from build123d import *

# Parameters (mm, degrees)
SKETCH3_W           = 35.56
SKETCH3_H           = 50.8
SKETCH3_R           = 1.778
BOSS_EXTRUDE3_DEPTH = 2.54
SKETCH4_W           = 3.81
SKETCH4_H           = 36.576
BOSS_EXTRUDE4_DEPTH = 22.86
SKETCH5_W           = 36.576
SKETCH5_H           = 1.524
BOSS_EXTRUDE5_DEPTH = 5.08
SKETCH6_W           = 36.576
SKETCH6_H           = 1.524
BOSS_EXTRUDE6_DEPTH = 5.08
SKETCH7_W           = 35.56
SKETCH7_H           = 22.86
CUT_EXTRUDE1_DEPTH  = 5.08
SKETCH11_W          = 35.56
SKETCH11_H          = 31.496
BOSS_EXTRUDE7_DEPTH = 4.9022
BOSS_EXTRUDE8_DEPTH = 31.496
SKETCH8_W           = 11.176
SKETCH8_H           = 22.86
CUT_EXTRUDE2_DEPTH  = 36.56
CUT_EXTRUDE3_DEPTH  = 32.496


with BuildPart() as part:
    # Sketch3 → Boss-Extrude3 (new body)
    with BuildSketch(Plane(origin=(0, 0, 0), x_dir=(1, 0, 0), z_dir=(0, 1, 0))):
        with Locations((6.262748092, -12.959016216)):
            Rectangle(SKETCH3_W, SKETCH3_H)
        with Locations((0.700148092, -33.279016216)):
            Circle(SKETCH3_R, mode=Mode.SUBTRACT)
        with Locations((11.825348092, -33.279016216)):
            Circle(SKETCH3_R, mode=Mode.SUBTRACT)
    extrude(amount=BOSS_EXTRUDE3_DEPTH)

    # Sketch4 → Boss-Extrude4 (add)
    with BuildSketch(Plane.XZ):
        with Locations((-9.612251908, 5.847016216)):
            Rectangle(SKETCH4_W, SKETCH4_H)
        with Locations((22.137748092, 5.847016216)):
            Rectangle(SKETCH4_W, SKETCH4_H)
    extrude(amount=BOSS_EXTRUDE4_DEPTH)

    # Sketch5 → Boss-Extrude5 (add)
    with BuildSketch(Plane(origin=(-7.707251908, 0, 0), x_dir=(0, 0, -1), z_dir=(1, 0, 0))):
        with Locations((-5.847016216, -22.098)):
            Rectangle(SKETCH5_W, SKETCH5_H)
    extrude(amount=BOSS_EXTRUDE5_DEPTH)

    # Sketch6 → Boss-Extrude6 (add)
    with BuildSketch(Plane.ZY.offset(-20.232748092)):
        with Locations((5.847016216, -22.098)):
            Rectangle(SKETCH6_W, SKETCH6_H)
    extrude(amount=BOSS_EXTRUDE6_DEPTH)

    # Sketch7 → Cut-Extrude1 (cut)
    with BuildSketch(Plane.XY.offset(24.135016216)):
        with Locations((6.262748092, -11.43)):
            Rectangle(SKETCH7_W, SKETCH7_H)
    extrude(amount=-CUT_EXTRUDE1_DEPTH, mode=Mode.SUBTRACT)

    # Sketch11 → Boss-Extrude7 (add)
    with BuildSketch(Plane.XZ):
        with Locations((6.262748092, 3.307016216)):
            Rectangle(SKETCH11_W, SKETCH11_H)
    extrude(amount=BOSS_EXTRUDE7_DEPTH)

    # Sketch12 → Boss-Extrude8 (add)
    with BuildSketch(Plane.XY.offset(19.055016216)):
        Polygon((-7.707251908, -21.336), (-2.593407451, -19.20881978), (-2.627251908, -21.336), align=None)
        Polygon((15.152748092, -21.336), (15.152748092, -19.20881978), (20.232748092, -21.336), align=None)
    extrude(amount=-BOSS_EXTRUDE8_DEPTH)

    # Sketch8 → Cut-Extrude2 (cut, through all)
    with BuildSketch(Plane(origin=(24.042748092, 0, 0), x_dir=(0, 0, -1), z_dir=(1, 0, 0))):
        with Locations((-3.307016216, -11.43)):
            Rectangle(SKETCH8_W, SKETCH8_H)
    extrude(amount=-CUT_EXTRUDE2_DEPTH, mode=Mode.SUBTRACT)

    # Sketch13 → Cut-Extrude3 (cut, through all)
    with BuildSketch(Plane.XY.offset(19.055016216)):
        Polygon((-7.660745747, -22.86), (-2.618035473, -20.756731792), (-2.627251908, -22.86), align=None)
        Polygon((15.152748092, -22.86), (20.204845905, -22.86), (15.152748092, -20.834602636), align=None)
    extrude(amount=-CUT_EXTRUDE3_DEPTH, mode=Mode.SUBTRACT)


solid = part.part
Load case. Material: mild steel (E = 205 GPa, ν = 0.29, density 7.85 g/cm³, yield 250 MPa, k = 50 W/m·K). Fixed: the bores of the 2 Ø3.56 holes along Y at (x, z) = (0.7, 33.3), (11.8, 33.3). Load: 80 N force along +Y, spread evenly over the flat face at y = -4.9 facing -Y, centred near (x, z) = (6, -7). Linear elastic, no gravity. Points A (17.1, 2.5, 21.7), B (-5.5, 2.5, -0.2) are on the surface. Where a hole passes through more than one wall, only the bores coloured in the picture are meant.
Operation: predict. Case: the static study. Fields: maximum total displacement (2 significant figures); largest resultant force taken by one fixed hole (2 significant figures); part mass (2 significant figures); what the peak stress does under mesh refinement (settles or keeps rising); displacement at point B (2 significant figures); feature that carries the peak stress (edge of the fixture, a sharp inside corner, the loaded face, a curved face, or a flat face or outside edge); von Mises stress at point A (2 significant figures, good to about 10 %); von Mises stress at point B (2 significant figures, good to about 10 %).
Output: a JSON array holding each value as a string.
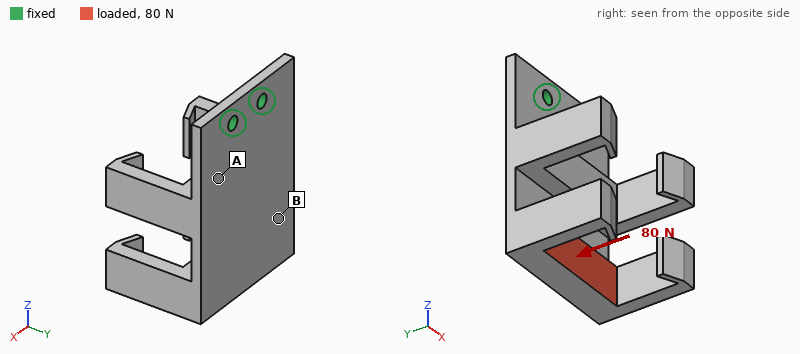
["0.21 mm", "40 N", "88 g", "keeps rising", "0.11 mm", "edge of the fixture", "55 MPa", "14 MPa"]
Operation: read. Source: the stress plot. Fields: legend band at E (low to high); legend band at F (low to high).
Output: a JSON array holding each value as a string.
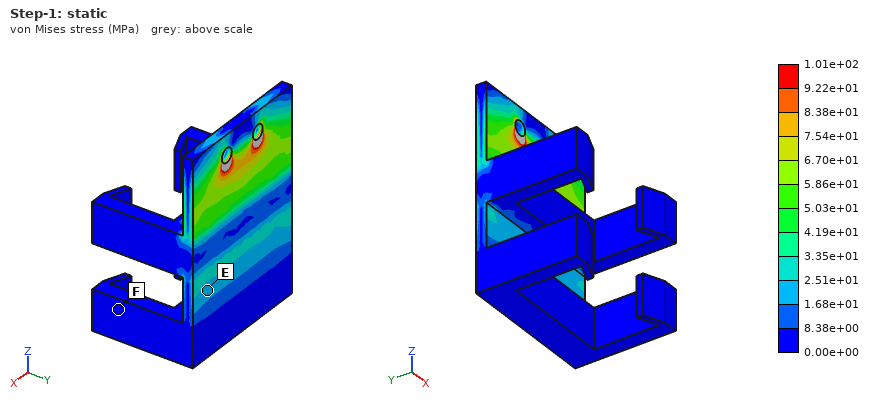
["1.68e+01 to 2.51e+01 MPa", "0.00e+00 to 8.38e+00 MPa"]
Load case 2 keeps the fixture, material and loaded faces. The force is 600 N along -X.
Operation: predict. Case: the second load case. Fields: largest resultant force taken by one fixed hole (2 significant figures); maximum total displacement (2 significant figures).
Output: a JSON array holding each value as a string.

["1.7 kN", "0.10 mm"]
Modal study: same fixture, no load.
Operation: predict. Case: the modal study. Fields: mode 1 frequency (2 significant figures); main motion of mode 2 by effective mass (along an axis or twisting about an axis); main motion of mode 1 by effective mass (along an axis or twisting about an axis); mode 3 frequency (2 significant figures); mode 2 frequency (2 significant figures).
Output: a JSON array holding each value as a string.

["530 Hz", "along X", "along Y", "2500 Hz", "1500 Hz"]
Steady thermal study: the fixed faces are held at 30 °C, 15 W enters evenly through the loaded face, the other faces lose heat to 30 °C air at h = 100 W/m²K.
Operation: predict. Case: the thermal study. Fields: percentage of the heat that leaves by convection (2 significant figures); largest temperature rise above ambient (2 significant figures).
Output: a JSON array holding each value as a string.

["82 %", "44 K"]
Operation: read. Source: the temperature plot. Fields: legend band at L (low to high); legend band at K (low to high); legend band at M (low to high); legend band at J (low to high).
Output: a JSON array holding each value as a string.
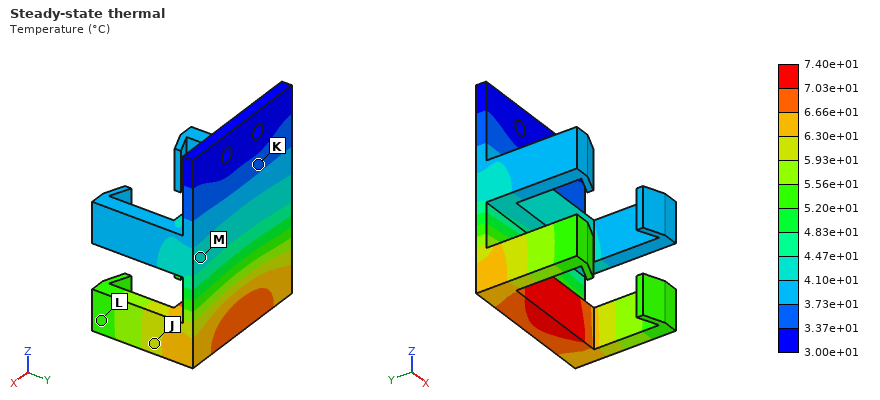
["5.20e+01 to 5.56e+01 °C", "3.37e+01 to 3.73e+01 °C", "4.10e+01 to 4.47e+01 °C", "5.93e+01 to 6.30e+01 °C"]
